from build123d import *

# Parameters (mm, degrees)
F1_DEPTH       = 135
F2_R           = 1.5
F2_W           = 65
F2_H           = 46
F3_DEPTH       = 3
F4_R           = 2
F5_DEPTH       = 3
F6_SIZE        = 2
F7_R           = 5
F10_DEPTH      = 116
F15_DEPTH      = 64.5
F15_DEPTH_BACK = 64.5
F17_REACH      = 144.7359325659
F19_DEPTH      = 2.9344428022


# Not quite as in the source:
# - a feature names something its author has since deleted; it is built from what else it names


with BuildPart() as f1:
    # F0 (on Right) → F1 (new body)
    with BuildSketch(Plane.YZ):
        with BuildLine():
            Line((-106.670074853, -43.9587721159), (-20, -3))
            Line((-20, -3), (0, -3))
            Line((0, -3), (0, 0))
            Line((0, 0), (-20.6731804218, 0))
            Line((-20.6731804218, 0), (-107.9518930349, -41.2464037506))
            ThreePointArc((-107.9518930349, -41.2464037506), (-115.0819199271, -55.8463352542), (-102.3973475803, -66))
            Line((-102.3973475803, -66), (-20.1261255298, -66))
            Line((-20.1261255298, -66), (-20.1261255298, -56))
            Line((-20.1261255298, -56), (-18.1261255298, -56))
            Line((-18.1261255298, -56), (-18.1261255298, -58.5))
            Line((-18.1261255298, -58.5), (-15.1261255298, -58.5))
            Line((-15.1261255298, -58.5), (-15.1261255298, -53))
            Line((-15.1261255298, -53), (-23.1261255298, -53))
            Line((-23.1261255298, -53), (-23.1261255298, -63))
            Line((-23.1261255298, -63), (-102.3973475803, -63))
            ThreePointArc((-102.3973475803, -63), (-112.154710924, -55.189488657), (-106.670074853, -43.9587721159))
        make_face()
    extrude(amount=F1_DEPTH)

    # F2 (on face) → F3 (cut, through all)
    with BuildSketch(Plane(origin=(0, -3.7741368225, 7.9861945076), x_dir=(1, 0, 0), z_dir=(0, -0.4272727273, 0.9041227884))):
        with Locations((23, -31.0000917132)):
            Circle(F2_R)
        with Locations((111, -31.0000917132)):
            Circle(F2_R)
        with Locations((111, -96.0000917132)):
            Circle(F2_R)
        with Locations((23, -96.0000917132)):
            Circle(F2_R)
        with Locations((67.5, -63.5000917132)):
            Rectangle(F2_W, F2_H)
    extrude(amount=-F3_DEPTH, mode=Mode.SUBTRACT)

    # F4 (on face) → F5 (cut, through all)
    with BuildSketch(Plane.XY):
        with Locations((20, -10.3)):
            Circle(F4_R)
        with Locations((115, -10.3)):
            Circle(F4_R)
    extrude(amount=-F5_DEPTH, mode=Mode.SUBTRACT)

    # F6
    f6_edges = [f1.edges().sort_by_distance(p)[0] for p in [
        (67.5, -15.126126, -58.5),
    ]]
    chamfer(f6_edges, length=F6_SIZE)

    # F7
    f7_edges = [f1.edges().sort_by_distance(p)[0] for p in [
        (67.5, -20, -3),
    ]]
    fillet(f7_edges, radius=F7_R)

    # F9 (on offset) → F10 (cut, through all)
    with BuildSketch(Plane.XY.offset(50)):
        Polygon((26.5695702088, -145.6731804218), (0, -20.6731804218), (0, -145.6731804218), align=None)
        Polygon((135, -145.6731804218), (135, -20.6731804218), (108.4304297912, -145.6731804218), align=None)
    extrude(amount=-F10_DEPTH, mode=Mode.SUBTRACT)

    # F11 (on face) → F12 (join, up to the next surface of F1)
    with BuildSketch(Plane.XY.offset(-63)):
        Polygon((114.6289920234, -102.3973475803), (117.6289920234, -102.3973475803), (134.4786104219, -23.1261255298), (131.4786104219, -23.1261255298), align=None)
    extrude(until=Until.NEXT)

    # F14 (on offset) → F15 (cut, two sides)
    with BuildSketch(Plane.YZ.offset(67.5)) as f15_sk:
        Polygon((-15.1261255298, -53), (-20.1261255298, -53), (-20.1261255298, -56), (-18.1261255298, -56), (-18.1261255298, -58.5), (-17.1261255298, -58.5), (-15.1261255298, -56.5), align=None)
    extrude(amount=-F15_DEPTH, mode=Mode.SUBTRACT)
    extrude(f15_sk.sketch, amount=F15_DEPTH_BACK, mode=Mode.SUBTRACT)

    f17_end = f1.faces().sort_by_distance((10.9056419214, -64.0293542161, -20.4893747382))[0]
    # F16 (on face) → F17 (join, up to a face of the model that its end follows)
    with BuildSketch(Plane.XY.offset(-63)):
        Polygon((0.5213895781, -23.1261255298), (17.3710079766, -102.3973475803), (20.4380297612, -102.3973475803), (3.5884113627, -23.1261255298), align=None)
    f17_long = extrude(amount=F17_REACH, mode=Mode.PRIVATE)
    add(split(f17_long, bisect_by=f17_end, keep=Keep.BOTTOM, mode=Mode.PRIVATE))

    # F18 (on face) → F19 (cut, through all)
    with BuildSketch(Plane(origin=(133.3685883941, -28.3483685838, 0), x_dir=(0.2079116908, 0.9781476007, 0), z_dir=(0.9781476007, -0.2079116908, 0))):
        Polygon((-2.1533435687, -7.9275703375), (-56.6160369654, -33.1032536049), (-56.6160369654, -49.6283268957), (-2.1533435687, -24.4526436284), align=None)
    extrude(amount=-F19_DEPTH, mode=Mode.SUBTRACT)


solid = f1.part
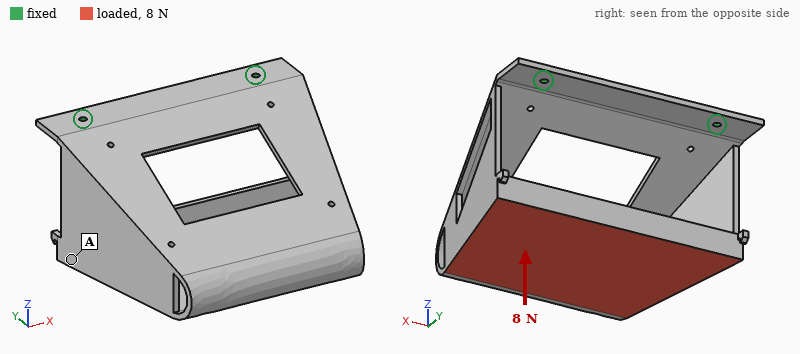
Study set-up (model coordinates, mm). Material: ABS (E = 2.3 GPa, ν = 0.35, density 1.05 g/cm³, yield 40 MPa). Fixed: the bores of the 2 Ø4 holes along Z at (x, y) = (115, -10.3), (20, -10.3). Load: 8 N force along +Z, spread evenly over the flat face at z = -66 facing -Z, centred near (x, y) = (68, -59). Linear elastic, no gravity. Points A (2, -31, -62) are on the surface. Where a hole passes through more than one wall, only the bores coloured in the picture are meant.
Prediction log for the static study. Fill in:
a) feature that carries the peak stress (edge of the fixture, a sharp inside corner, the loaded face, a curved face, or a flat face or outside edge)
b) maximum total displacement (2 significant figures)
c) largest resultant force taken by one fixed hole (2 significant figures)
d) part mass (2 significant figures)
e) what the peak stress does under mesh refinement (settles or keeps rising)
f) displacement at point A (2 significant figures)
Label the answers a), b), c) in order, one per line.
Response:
a) edge of the fixture
b) 2.0 mm
c) 4.1 N
d) 96 g
e) keeps rising
f) 1.1 mm
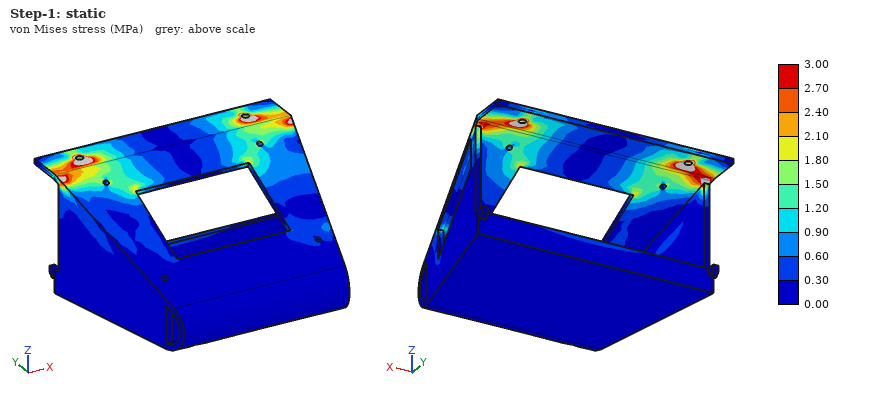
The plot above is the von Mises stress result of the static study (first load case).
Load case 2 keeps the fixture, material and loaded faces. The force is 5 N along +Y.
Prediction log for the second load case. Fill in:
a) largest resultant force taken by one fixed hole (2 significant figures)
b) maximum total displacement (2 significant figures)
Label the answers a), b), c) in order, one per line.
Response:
a) 2.6 N
b) 2.1 mm
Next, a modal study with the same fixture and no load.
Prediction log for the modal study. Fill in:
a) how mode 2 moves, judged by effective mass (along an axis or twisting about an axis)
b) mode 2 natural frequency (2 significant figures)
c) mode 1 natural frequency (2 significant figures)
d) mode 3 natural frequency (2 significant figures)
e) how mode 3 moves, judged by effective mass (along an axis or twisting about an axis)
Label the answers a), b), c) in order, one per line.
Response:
a) along X
b) 100 Hz
c) 31 Hz
d) 290 Hz
e) along Z
